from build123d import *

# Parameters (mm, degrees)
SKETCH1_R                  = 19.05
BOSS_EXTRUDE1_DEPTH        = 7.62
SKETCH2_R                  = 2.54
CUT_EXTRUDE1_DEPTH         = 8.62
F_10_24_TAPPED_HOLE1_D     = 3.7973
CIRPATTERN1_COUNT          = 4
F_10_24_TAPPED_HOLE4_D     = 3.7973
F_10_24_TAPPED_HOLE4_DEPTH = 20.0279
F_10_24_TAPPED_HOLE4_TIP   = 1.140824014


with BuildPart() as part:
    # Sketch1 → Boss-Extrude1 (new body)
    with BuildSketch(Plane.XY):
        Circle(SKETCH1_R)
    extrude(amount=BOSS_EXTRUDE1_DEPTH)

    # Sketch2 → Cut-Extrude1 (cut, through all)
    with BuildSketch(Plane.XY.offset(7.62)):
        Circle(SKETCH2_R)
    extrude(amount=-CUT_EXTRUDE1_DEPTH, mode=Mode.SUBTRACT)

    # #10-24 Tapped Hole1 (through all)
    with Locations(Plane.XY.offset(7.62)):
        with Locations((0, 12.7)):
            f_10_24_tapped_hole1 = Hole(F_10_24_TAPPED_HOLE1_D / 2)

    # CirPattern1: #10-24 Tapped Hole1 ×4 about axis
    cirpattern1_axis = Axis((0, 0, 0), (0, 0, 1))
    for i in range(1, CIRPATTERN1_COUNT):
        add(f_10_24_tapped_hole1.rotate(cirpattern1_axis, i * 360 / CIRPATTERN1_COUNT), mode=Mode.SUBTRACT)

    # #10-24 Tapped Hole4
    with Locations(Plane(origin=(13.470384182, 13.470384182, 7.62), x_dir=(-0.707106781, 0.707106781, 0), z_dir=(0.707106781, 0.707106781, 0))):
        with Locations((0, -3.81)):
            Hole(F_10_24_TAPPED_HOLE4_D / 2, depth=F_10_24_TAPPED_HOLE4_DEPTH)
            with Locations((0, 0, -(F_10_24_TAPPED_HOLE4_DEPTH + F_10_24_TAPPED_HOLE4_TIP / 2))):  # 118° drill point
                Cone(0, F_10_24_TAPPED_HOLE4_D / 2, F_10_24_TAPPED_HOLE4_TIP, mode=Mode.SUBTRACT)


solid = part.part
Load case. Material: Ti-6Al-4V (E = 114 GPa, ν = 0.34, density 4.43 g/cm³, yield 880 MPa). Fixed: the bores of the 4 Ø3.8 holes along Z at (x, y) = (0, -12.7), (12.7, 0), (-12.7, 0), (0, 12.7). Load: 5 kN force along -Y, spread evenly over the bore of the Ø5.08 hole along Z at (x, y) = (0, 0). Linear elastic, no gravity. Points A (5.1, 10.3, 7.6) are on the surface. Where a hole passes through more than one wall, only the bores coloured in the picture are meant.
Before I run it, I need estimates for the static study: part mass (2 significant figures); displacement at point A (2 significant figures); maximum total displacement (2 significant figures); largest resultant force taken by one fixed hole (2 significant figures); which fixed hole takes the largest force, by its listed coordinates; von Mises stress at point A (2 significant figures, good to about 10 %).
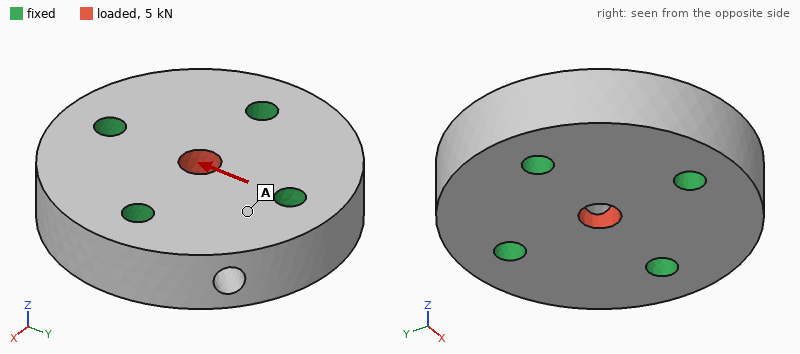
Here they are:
35 g
0.70 µm
3.1 µm
1.8 kN
(0, -12.7)
8.6 MPa
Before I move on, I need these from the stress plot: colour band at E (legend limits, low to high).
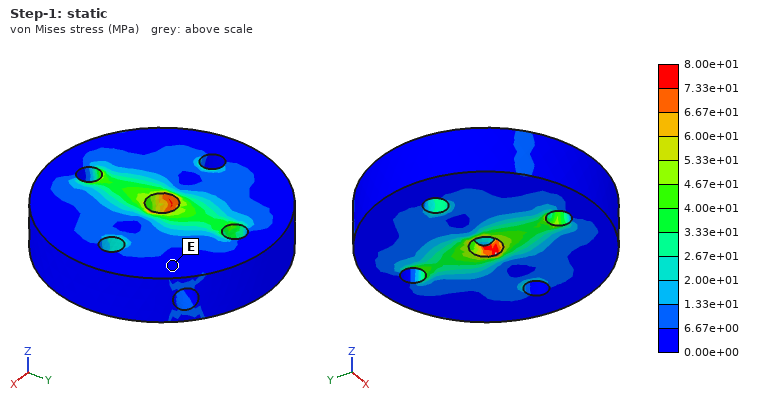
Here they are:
0.00e+00 to 6.67e+00 MPa
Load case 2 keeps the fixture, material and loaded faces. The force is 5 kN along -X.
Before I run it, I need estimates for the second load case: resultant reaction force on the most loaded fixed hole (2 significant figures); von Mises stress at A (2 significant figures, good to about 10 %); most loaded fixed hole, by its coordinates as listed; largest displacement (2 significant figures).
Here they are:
1.8 kN
8.0 MPa
(-12.7, 0)
3.1 µm
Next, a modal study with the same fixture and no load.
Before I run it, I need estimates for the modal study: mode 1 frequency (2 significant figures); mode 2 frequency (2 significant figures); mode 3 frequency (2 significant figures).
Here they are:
47 kHz
48 kHz
50 kHz
